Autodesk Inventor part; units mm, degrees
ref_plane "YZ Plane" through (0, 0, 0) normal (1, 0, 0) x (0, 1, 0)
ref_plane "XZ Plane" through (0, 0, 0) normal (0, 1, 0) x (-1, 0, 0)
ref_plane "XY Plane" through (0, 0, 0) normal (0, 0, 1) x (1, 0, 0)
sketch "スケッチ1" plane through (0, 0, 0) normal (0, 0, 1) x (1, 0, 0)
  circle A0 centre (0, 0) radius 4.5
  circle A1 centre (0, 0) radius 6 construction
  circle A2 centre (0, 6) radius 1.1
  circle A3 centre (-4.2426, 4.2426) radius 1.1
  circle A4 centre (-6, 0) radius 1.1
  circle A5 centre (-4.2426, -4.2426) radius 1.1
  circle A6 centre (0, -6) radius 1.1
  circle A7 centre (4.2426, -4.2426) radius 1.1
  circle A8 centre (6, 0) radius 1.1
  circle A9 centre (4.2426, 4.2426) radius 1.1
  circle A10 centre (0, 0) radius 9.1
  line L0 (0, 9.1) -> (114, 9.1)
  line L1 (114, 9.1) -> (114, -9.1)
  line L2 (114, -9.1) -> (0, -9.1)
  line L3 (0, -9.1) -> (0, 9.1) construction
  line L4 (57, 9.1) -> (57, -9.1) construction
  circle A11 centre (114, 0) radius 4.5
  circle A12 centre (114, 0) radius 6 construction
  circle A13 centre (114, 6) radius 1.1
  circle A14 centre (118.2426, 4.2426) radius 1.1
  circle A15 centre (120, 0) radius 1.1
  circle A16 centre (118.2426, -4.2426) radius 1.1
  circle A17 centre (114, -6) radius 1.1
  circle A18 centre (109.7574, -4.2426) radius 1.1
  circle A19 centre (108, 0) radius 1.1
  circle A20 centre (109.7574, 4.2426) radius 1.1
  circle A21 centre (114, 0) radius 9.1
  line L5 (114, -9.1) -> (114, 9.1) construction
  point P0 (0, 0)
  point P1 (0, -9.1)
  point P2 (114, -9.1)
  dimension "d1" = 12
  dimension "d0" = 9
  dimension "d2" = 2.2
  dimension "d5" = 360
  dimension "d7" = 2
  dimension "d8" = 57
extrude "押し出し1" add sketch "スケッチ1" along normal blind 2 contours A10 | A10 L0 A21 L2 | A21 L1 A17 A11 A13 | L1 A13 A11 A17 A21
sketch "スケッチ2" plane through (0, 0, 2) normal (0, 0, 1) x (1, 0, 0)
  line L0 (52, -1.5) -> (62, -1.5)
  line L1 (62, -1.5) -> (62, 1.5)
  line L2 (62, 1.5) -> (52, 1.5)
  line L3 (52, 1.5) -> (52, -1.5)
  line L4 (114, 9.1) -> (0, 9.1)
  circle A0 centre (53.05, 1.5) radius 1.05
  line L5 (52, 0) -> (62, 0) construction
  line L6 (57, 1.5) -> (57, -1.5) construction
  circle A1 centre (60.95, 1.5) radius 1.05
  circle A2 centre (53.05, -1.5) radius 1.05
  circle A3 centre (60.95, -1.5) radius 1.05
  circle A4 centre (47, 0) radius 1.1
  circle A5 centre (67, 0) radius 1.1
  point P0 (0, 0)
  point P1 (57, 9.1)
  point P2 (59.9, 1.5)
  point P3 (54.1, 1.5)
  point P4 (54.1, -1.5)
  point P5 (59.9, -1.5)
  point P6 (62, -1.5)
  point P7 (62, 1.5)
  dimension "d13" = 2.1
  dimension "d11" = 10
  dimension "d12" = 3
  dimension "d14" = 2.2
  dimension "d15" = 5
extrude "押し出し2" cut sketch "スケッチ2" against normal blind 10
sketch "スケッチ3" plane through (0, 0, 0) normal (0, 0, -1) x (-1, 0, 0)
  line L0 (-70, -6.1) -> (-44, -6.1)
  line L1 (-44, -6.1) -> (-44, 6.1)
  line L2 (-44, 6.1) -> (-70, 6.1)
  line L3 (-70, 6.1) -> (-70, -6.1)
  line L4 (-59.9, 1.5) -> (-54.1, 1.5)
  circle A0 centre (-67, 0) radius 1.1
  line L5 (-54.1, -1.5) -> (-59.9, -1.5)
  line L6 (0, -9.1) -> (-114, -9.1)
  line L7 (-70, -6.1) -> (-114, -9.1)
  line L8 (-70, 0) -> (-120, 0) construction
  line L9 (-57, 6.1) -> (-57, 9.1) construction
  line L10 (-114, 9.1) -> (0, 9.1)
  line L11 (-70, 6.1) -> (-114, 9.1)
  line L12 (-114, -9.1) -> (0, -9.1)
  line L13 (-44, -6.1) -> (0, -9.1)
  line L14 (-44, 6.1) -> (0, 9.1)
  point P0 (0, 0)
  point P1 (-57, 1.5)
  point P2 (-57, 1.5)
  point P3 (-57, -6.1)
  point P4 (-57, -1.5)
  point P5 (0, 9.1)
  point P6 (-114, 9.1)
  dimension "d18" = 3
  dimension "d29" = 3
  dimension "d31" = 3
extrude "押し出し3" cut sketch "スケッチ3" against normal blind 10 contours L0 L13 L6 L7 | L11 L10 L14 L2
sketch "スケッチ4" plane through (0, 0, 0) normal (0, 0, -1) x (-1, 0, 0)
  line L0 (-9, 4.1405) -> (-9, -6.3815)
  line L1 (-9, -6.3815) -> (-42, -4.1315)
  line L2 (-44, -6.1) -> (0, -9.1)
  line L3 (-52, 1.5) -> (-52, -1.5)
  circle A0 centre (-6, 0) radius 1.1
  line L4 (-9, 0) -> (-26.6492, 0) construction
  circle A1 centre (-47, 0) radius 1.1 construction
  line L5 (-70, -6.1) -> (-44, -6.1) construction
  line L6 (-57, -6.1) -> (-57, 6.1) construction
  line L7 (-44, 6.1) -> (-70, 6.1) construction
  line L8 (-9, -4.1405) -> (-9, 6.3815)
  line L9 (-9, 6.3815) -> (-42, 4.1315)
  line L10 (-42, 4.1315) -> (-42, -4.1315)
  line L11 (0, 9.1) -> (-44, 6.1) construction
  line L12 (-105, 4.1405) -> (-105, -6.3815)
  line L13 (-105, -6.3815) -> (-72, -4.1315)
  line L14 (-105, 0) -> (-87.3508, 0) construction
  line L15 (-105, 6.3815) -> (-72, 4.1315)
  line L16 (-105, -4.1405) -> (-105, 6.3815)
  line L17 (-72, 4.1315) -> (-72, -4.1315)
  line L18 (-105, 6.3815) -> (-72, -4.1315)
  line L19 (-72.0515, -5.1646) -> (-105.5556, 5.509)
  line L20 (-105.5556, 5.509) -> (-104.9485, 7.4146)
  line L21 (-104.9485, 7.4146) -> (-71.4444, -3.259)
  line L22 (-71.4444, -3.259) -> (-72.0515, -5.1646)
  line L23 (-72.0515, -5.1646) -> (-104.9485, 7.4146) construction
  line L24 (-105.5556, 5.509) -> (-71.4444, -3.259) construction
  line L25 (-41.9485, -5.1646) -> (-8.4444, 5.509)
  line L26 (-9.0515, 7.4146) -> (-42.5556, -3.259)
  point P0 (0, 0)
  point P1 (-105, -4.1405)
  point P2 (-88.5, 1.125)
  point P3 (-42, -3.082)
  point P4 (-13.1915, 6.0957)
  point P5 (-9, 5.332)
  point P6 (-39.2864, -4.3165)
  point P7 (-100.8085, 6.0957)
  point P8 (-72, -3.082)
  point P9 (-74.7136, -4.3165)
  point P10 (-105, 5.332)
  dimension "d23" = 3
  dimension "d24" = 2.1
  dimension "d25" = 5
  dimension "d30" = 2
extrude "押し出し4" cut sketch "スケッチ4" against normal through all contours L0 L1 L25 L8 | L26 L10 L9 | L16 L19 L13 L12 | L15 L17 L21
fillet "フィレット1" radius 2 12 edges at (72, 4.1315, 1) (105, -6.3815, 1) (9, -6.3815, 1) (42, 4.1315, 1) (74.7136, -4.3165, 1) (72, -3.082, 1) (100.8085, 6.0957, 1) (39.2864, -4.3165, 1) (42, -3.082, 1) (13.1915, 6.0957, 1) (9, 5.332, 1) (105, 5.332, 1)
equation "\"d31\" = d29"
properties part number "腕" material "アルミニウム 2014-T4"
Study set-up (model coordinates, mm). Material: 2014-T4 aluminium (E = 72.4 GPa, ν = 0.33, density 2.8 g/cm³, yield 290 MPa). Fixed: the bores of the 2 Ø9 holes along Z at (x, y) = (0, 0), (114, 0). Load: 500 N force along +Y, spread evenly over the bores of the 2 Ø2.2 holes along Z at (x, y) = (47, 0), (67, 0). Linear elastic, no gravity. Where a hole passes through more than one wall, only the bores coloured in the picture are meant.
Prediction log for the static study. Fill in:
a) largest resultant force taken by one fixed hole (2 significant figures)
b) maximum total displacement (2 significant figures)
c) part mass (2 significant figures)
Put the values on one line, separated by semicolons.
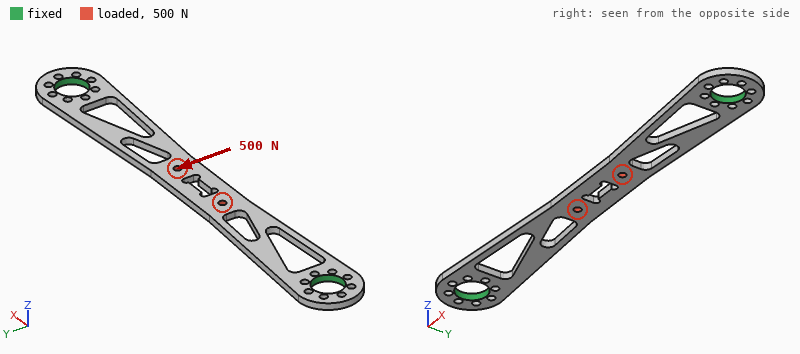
300 N; 0.25 mm; 6.8 g
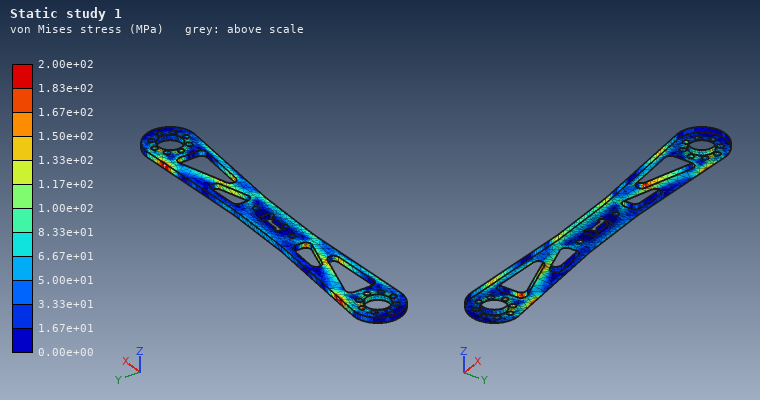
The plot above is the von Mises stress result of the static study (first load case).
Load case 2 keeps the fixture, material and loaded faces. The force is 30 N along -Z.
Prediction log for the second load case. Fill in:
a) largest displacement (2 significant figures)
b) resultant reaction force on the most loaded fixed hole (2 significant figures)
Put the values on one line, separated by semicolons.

0.44 mm; 15 N
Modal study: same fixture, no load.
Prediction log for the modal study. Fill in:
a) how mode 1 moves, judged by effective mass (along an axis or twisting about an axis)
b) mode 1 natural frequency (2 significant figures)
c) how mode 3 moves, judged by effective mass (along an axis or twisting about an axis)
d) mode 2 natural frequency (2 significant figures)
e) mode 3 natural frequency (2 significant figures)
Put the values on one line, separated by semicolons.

along Z; 850 Hz; twisting about X; 2400 Hz; 3300 Hz
